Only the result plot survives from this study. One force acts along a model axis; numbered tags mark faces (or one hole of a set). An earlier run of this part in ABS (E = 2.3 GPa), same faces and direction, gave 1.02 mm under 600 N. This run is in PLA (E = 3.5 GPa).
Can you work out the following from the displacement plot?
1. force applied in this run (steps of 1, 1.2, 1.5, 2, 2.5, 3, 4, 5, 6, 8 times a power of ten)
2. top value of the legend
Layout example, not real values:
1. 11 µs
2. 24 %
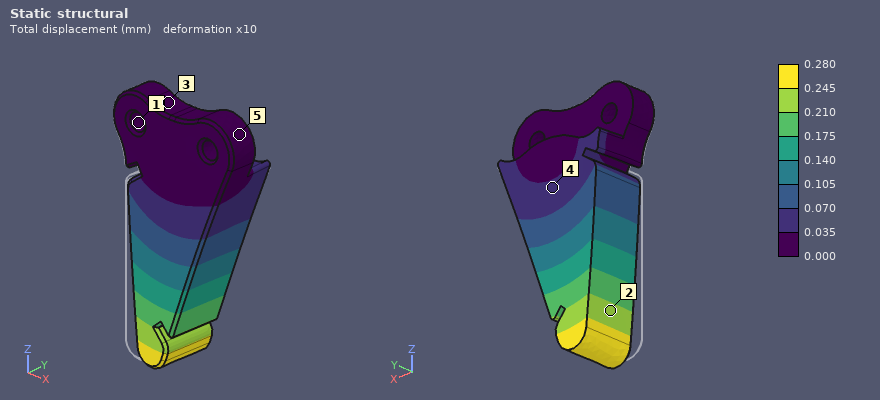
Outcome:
1. 250 N
2. 0.280 mm
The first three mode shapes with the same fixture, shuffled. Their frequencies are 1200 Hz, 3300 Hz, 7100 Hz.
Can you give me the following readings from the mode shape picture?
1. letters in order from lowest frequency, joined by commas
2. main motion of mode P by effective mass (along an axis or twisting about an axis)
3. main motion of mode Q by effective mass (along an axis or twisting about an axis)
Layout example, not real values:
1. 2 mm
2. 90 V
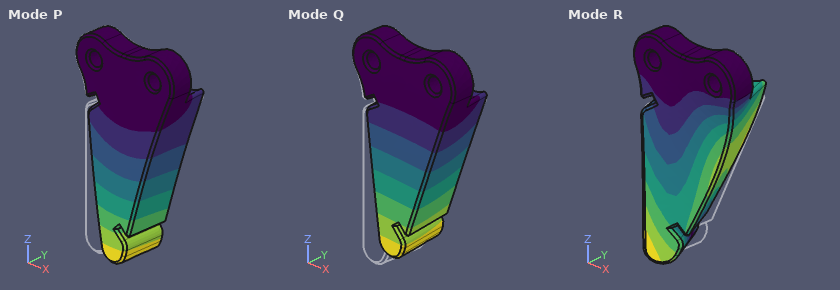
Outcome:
1. Q, P, R
2. along X
3. along Y
